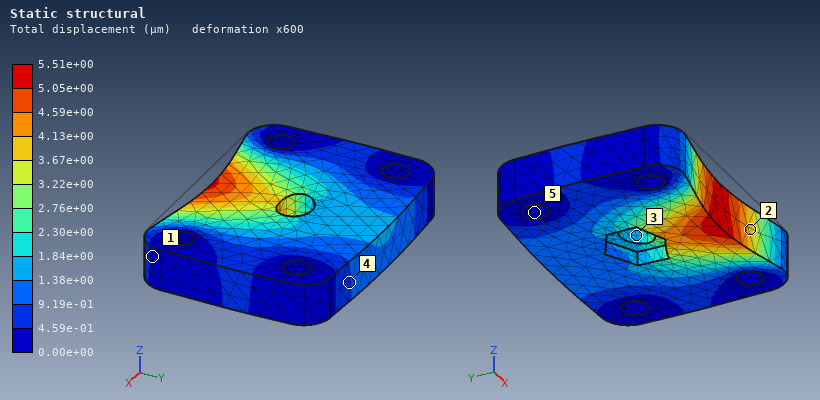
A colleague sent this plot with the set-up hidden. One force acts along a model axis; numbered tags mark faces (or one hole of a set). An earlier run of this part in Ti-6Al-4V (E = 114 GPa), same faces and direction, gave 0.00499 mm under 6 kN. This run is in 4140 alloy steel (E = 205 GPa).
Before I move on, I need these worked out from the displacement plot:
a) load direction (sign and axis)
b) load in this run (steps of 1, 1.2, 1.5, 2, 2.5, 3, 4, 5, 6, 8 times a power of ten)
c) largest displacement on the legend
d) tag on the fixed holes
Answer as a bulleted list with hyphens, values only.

- +Y
- 12 kN
- 5.51e+00 µm
- 5
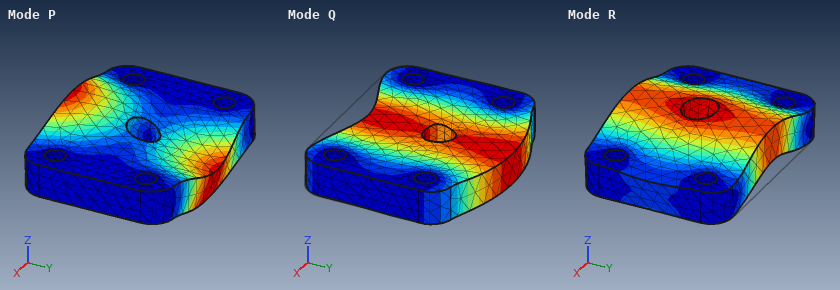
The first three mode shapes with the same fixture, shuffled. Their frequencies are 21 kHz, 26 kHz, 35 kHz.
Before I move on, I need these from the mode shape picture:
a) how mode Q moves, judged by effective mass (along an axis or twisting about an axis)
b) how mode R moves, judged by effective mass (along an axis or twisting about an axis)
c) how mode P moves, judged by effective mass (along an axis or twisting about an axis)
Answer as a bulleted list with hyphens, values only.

- along Y
- along Z
- twisting about X
